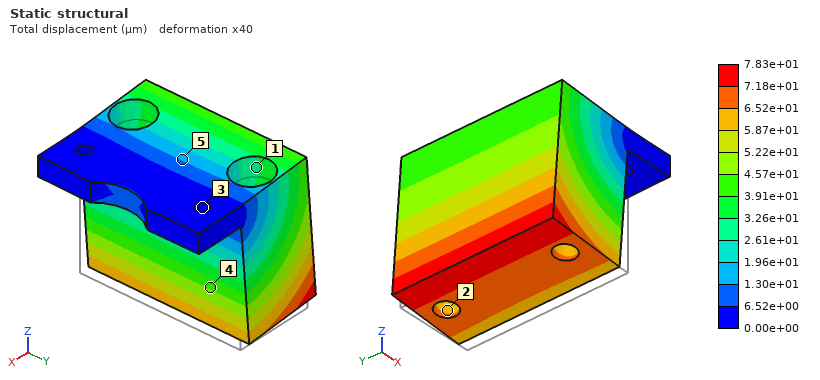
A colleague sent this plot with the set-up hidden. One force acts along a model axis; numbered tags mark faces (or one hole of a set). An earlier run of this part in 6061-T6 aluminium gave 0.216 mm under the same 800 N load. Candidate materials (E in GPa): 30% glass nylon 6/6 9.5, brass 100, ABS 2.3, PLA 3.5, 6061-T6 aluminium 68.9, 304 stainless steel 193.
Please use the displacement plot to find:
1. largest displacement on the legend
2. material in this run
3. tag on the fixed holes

7.83e+01 µm
304 stainless steel
3
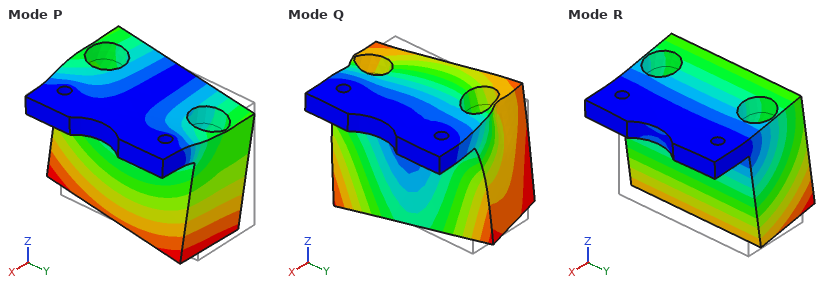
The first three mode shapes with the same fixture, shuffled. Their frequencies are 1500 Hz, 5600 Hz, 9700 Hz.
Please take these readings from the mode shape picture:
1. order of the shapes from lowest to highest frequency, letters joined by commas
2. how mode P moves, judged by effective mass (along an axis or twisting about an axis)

R, P, Q
along Y
